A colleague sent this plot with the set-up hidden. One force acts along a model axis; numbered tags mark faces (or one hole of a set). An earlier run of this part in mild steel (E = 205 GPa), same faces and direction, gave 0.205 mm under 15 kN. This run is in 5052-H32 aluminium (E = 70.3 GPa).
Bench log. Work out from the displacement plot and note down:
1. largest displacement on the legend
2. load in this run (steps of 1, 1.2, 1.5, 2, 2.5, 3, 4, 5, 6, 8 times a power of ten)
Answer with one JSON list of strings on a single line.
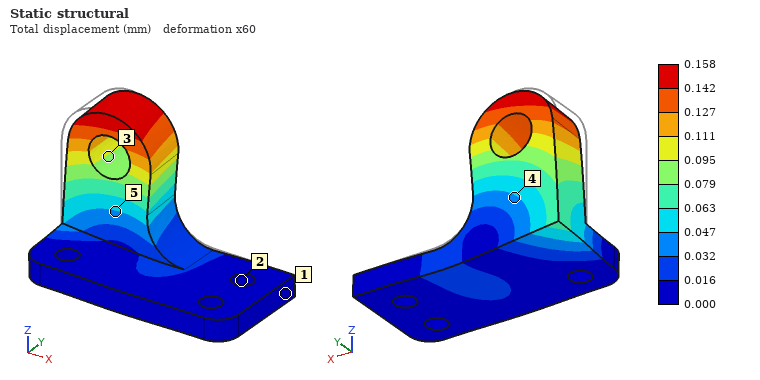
["0.158 mm", "4 kN"]
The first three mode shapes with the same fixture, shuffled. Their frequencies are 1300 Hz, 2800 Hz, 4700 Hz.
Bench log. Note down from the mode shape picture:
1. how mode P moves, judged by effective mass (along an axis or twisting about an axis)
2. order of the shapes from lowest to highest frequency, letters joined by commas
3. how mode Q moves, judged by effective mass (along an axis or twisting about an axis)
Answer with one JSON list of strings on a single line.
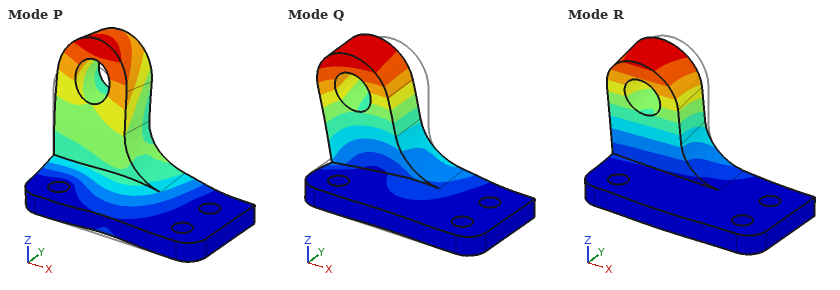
["along Z", "R, Q, P", "along X"]
